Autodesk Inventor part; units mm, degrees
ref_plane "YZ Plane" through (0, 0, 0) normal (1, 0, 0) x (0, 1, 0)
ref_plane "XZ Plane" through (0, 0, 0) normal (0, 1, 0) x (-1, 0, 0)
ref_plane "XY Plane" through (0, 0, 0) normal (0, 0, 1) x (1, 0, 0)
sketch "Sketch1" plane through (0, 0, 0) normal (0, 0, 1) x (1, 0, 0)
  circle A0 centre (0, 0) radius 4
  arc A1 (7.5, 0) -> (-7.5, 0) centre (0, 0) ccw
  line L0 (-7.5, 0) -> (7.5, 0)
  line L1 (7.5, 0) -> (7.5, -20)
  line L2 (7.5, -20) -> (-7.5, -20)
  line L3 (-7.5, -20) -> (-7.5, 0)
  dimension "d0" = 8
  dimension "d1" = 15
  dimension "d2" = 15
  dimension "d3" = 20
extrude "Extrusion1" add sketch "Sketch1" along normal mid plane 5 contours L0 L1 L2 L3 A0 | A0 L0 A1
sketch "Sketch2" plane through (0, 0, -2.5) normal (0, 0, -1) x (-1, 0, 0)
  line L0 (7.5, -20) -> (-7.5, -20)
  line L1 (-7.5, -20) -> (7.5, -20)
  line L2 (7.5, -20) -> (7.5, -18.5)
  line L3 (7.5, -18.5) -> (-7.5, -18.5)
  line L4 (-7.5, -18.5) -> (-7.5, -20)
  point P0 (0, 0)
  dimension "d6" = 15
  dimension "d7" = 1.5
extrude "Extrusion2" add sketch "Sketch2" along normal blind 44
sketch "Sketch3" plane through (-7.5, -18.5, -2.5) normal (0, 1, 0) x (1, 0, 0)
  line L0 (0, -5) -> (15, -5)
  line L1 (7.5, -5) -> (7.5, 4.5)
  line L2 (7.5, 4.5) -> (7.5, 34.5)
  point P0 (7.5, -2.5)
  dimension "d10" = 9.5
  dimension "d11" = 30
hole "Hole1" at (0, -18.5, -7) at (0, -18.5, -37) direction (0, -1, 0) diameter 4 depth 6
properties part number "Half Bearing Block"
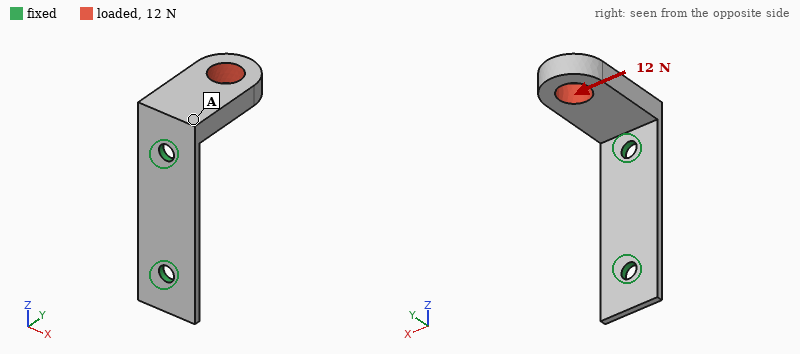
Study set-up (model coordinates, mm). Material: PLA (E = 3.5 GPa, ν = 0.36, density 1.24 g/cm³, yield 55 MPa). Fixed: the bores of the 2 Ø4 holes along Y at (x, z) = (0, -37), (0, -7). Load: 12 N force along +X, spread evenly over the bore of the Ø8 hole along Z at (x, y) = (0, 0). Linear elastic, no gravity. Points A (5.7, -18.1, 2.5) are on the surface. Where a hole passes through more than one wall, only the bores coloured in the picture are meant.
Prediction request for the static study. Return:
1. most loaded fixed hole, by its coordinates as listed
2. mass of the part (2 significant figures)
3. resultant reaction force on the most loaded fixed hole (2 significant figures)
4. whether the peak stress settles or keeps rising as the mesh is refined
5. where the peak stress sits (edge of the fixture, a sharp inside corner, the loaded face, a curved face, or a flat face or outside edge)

(0, -7)
3.3 g
13 N
keeps rising
edge of the fixture
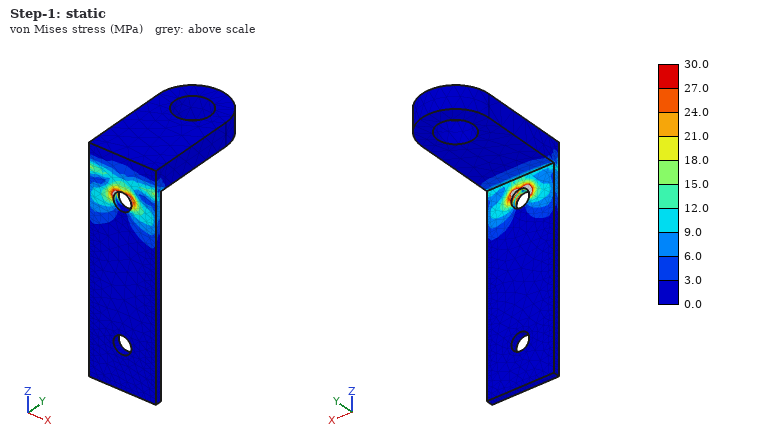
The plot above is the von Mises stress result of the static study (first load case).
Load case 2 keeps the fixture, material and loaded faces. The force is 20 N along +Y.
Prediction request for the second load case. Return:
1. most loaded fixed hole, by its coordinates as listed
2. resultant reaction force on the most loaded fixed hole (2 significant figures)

(0, -7)
20 N
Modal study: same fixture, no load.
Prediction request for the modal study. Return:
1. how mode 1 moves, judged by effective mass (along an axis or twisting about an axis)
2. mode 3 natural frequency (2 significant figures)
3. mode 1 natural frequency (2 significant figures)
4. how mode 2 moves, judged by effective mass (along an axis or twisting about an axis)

along Z
3200 Hz
470 Hz
along X
